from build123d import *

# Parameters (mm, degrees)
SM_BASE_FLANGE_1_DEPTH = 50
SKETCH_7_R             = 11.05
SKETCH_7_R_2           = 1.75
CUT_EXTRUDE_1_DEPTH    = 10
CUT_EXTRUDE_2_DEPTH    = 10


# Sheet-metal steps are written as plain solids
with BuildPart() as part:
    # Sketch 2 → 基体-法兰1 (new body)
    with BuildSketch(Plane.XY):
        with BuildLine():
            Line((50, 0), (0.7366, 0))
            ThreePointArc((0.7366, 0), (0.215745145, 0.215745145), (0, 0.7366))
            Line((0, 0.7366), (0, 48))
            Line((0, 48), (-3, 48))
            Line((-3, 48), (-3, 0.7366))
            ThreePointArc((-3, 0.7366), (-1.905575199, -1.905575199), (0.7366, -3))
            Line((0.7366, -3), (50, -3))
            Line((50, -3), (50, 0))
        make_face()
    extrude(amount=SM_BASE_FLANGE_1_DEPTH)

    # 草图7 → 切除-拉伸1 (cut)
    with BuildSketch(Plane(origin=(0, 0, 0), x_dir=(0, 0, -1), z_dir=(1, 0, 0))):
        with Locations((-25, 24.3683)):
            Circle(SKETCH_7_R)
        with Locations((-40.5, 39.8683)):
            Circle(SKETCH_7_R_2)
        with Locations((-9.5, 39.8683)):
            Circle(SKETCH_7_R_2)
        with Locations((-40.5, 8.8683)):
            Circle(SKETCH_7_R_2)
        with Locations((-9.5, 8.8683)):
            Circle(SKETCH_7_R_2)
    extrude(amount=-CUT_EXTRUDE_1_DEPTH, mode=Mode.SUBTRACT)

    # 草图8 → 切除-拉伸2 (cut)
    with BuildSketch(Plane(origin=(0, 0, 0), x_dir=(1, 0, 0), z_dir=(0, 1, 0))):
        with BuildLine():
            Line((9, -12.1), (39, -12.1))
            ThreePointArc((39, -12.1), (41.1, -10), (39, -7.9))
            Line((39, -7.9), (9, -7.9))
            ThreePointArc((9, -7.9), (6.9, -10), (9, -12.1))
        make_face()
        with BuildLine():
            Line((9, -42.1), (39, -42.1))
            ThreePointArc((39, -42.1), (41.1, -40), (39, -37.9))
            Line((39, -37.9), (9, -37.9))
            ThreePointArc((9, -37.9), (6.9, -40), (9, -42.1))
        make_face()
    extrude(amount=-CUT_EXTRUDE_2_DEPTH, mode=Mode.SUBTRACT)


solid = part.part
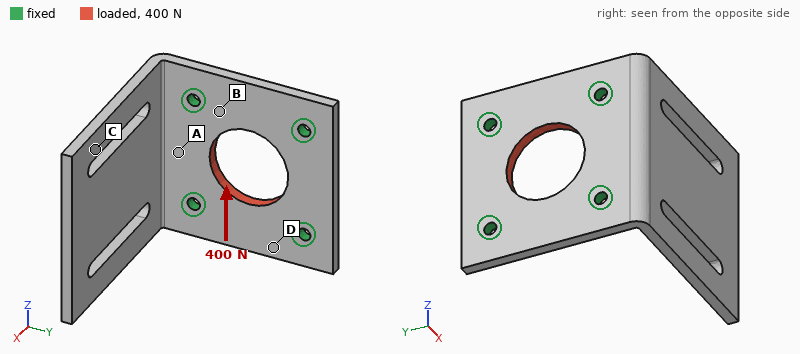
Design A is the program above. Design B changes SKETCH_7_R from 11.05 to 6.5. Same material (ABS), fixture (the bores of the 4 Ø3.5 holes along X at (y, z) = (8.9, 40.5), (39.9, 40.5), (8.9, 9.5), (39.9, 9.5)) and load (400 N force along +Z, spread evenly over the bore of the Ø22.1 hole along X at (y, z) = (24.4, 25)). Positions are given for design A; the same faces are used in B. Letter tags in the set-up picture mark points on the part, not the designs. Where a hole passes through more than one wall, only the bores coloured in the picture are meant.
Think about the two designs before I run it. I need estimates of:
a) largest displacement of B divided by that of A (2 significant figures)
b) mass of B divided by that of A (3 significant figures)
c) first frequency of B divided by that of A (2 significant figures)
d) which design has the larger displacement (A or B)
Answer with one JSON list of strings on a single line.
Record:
["1.1", "1.06", "1.0", "B"]
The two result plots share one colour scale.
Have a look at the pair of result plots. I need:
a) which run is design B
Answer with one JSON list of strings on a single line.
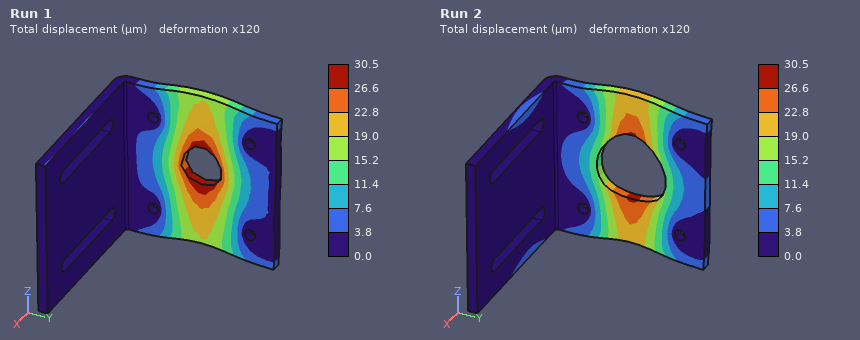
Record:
["Run 1"]
